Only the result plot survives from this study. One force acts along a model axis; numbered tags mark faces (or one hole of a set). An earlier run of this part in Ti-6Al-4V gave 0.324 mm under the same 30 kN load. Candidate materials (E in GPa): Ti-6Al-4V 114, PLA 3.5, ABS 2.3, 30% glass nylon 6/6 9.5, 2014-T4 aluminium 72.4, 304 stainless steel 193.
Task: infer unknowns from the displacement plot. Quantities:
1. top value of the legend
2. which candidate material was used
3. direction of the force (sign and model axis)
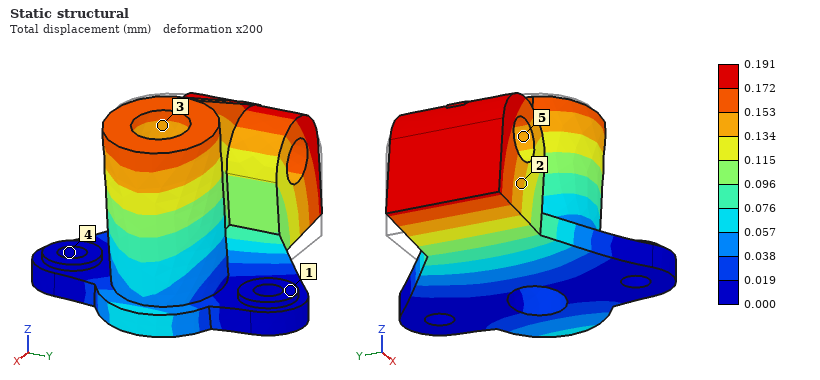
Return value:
0.191 mm
304 stainless steel
+X
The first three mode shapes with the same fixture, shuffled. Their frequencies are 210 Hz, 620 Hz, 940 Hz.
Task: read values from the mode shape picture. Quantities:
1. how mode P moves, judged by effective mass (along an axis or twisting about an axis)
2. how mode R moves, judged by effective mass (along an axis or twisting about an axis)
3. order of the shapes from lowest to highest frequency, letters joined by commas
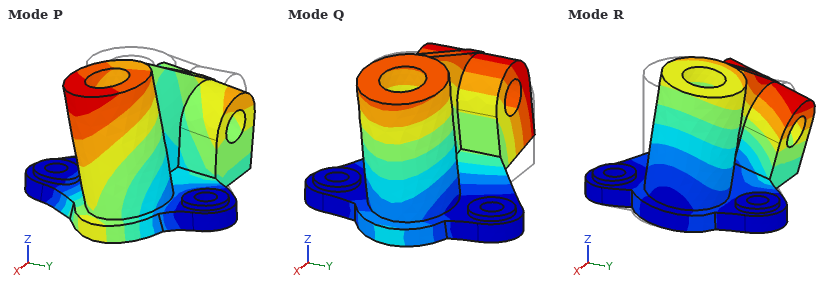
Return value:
along Z
along Y
Q, R, P
